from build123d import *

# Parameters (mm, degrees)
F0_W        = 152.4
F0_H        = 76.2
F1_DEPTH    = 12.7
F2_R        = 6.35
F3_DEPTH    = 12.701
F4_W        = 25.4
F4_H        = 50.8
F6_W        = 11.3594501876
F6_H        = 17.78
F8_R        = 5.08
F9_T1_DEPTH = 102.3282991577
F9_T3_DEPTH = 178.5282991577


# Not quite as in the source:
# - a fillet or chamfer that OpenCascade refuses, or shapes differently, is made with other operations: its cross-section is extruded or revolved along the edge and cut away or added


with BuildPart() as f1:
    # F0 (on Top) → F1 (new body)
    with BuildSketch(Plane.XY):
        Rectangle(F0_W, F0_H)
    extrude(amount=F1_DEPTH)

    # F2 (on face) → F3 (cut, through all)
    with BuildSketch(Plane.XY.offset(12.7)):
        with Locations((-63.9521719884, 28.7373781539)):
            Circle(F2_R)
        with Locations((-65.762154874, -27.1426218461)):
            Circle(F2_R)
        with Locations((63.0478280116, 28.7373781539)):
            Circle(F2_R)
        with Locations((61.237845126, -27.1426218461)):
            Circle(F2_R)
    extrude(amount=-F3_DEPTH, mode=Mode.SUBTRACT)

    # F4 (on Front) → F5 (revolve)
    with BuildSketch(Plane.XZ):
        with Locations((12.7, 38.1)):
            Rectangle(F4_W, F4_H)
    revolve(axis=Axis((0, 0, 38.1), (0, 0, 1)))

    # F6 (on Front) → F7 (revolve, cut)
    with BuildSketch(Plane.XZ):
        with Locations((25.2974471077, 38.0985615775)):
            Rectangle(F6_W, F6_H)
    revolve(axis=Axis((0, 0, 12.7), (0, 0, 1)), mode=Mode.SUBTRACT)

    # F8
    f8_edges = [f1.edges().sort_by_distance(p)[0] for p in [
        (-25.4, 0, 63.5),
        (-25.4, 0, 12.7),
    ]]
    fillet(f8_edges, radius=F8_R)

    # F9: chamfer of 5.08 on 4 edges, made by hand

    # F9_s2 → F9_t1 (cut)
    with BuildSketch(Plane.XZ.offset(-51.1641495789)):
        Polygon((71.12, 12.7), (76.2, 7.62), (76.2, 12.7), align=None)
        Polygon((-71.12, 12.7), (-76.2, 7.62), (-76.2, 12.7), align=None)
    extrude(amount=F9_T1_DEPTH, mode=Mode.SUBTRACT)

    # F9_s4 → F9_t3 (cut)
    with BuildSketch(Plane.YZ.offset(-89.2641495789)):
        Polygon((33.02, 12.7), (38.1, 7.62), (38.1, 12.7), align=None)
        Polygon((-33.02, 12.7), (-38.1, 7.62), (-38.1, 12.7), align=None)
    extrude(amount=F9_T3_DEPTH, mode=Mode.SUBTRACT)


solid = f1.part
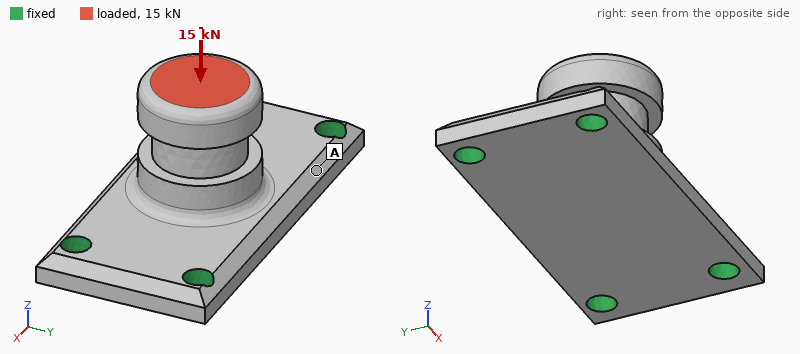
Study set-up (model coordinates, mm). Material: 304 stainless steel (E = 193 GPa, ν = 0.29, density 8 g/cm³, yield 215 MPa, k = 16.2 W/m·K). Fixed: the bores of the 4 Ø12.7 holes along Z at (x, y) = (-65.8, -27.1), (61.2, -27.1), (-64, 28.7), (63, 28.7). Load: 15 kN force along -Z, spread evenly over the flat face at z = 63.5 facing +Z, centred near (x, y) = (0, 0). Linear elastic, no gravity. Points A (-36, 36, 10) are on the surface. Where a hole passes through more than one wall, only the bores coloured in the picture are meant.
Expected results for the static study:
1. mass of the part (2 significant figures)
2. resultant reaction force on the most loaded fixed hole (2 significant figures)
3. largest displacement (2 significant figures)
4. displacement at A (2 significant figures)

1.8 kg
4.5 kN
36 µm
17 µm
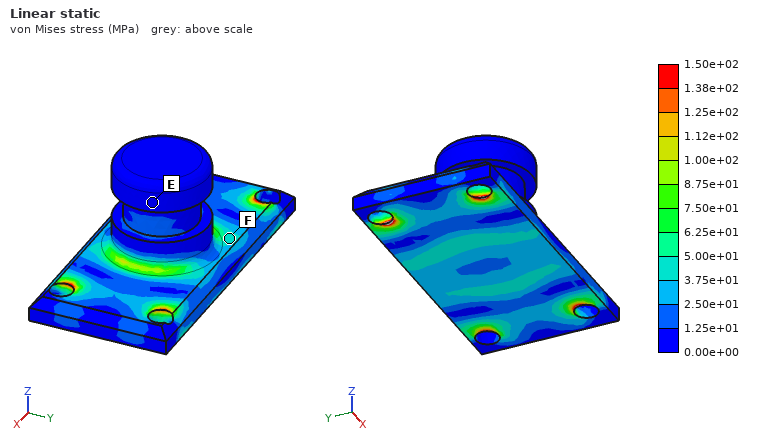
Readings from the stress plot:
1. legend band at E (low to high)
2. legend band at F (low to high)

0.00e+00 to 1.25e+01 MPa
3.75e+01 to 5.00e+01 MPa
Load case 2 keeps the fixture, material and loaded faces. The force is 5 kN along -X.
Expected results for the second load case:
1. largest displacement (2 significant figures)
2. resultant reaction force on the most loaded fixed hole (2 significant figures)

29 µm
2.1 kN
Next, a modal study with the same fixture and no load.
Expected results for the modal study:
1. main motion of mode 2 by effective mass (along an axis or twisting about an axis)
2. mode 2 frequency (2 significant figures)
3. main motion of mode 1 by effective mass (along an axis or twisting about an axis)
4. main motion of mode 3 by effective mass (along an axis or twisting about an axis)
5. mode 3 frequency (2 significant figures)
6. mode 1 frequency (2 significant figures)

along Z
3100 Hz
along Y
along X
4100 Hz
2500 Hz
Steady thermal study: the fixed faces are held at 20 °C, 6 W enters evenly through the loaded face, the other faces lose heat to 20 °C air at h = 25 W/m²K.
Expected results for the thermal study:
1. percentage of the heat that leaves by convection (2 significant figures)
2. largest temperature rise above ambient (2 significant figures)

57 %
15 K
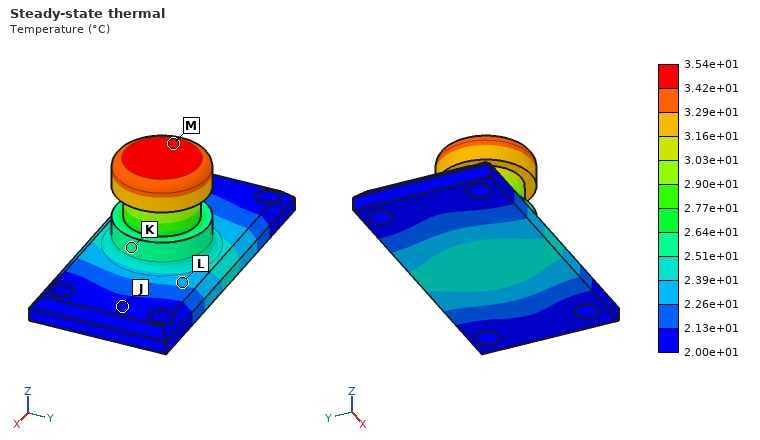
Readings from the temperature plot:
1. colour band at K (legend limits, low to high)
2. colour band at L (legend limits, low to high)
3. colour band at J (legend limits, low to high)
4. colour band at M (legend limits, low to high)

2.51e+01 to 2.64e+01 °C
2.26e+01 to 2.39e+01 °C
2.00e+01 to 2.13e+01 °C
3.42e+01 to 3.54e+01 °C
